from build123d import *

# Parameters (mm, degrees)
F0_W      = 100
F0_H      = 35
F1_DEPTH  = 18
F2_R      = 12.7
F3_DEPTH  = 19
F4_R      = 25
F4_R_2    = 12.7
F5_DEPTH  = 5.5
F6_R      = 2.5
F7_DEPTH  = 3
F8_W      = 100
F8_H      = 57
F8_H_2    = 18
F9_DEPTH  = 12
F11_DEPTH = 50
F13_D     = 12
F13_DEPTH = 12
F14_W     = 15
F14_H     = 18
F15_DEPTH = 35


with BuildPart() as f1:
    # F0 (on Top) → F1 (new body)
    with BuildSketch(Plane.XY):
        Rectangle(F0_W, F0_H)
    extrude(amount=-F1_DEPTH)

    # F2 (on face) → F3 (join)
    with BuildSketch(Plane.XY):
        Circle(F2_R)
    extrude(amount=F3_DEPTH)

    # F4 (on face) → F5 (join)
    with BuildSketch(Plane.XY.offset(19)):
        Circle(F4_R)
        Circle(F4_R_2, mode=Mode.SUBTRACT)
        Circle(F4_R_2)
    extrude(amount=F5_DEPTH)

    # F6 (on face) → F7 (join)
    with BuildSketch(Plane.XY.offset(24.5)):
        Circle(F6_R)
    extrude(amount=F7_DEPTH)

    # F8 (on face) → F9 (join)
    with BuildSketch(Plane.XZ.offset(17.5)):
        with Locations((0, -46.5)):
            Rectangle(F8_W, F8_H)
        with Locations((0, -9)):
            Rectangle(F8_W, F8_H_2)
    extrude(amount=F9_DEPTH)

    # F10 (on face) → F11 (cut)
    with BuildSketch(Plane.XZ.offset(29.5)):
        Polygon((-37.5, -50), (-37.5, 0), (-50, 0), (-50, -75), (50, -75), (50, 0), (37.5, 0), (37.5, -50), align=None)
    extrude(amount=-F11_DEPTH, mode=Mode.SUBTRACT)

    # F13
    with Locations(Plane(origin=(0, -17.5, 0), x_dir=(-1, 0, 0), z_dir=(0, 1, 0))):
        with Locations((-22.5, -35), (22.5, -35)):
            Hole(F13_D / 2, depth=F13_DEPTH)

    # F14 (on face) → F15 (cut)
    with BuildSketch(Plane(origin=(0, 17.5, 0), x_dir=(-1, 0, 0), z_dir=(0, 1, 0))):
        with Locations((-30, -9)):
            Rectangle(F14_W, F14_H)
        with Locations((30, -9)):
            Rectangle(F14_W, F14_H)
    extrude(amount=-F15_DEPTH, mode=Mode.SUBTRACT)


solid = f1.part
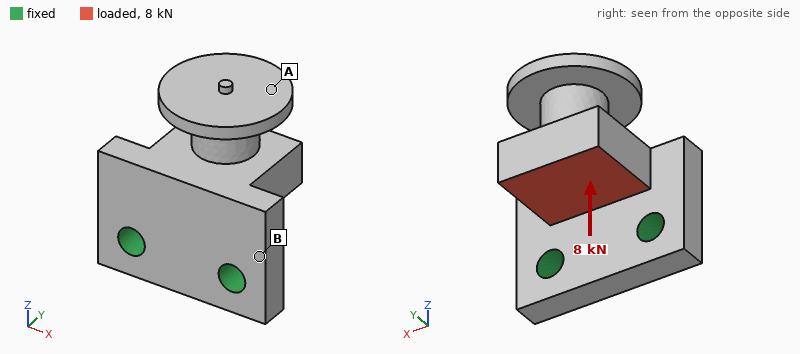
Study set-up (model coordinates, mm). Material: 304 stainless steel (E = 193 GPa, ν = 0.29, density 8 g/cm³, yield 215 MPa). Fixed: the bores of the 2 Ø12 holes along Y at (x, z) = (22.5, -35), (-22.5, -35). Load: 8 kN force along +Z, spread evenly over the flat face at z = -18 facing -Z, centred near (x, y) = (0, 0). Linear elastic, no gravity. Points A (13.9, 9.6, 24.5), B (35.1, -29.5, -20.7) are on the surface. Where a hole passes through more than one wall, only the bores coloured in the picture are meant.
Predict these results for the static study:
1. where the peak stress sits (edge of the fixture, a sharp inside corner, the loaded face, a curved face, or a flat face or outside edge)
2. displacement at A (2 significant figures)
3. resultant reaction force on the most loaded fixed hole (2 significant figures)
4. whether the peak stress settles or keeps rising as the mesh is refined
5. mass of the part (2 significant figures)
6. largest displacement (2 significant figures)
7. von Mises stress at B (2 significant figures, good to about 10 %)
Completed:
edge of the fixture
0.13 mm
4.2 kN
keeps rising
730 g
0.15 mm
78 MPa
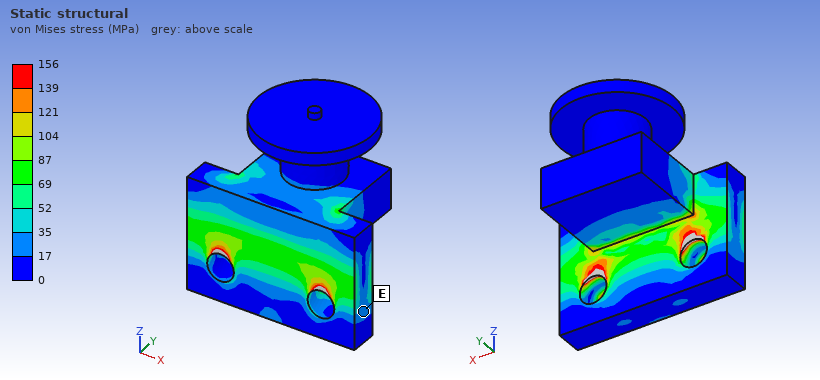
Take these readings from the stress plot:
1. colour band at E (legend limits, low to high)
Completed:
17 to 35 MPa
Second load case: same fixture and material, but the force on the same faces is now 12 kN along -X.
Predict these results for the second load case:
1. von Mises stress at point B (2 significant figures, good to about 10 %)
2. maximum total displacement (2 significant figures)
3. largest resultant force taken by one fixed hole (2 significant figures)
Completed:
23 MPa
49 µm
9.0 kN
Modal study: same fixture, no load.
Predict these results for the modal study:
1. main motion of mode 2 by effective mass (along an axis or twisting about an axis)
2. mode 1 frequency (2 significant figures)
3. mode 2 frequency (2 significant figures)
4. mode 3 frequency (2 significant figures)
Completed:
along X
1900 Hz
4800 Hz
6300 Hz
